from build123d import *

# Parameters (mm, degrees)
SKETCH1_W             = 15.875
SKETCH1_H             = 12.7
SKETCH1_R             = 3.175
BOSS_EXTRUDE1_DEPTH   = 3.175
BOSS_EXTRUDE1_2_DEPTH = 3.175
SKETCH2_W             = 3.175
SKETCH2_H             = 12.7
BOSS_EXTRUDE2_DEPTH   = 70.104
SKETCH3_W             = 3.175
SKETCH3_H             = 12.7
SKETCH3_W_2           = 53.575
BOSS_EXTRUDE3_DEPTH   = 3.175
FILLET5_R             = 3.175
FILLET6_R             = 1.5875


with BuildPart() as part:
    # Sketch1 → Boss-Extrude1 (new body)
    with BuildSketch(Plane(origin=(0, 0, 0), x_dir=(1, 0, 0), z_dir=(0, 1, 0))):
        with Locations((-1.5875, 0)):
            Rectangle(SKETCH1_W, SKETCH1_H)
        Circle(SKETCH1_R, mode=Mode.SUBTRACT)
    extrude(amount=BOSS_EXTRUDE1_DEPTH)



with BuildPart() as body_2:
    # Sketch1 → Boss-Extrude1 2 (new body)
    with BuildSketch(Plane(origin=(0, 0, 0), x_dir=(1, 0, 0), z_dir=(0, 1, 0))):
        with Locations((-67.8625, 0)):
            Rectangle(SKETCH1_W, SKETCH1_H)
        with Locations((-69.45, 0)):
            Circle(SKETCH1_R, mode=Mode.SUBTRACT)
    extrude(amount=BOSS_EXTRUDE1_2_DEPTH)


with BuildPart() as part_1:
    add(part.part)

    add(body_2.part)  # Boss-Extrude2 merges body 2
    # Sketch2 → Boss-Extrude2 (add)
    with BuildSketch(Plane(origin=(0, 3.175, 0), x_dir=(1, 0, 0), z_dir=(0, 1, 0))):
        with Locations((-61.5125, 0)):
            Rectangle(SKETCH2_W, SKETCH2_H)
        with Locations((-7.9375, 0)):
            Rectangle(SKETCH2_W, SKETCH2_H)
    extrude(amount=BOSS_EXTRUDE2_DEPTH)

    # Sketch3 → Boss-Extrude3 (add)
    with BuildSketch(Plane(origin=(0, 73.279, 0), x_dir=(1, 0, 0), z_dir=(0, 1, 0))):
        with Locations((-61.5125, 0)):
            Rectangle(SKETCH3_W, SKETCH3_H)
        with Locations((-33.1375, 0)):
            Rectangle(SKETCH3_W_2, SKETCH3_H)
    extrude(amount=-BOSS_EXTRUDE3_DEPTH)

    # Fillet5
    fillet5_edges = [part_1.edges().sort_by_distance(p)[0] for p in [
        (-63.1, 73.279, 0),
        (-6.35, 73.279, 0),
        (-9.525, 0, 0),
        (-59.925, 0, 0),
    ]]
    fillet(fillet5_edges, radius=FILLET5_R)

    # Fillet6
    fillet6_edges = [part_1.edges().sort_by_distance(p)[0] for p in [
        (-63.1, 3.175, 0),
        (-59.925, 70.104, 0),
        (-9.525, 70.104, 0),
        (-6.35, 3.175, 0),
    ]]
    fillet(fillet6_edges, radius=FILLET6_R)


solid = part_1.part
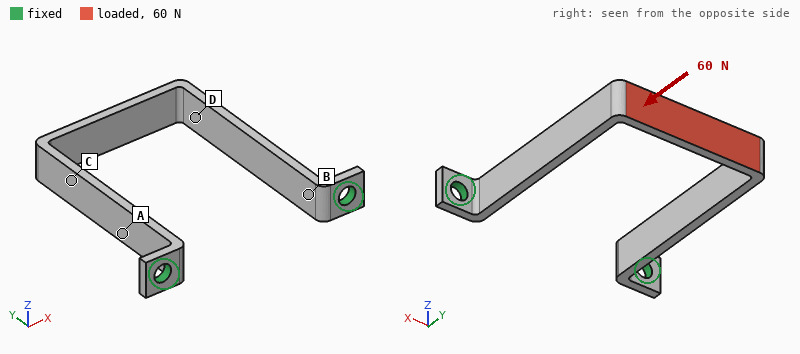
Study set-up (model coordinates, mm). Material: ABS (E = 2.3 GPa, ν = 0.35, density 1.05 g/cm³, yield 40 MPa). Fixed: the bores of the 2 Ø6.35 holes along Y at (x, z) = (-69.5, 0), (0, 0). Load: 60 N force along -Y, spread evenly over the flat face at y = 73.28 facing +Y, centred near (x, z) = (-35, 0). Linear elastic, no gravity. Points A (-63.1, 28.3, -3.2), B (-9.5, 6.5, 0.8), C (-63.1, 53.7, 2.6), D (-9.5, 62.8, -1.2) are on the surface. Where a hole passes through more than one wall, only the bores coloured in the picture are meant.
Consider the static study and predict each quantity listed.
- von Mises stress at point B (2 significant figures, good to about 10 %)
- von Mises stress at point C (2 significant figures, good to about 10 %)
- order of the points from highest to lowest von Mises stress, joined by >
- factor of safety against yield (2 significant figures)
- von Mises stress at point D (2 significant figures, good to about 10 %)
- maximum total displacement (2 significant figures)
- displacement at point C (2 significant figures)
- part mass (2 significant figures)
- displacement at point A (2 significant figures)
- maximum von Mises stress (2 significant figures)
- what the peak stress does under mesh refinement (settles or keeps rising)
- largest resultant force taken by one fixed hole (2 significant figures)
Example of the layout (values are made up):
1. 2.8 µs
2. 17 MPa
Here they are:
1. 2.6 MPa
2. 4.5 MPa
3. D > C > B > A
4. 3.4
5. 7.5 MPa
6. 0.84 mm
7. 0.39 mm
8. 9.1 g
9. 0.23 mm
10. 12 MPa
11. settles
12. 30 N
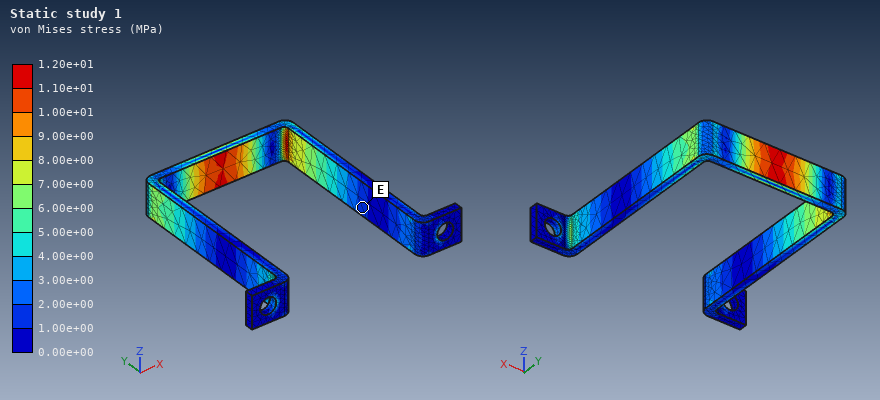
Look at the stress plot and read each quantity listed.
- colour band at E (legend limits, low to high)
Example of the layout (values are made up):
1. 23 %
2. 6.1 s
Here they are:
1. 1.00e+00 to 2.00e+00 MPa
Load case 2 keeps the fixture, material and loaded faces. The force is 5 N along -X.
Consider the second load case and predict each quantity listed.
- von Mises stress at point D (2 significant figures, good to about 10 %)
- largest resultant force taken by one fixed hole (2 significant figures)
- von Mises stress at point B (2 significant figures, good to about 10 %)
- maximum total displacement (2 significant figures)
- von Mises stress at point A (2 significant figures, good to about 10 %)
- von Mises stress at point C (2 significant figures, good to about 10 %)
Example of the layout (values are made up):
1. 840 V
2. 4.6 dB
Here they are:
1. 2.9 MPa
2. 4.1 N
3. 3.3 MPa
4. 1.3 mm
5. 1.2 MPa
6. 1.7 MPa
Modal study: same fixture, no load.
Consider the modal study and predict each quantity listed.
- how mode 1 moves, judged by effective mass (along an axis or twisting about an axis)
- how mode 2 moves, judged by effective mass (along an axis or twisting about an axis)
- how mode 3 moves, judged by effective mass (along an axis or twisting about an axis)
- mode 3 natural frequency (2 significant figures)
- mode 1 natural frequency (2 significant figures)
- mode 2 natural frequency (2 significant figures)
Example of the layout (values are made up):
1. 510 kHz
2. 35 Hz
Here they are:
1. along X
2. along Z
3. twisting about Y
4. 360 Hz
5. 150 Hz
6. 230 Hz
